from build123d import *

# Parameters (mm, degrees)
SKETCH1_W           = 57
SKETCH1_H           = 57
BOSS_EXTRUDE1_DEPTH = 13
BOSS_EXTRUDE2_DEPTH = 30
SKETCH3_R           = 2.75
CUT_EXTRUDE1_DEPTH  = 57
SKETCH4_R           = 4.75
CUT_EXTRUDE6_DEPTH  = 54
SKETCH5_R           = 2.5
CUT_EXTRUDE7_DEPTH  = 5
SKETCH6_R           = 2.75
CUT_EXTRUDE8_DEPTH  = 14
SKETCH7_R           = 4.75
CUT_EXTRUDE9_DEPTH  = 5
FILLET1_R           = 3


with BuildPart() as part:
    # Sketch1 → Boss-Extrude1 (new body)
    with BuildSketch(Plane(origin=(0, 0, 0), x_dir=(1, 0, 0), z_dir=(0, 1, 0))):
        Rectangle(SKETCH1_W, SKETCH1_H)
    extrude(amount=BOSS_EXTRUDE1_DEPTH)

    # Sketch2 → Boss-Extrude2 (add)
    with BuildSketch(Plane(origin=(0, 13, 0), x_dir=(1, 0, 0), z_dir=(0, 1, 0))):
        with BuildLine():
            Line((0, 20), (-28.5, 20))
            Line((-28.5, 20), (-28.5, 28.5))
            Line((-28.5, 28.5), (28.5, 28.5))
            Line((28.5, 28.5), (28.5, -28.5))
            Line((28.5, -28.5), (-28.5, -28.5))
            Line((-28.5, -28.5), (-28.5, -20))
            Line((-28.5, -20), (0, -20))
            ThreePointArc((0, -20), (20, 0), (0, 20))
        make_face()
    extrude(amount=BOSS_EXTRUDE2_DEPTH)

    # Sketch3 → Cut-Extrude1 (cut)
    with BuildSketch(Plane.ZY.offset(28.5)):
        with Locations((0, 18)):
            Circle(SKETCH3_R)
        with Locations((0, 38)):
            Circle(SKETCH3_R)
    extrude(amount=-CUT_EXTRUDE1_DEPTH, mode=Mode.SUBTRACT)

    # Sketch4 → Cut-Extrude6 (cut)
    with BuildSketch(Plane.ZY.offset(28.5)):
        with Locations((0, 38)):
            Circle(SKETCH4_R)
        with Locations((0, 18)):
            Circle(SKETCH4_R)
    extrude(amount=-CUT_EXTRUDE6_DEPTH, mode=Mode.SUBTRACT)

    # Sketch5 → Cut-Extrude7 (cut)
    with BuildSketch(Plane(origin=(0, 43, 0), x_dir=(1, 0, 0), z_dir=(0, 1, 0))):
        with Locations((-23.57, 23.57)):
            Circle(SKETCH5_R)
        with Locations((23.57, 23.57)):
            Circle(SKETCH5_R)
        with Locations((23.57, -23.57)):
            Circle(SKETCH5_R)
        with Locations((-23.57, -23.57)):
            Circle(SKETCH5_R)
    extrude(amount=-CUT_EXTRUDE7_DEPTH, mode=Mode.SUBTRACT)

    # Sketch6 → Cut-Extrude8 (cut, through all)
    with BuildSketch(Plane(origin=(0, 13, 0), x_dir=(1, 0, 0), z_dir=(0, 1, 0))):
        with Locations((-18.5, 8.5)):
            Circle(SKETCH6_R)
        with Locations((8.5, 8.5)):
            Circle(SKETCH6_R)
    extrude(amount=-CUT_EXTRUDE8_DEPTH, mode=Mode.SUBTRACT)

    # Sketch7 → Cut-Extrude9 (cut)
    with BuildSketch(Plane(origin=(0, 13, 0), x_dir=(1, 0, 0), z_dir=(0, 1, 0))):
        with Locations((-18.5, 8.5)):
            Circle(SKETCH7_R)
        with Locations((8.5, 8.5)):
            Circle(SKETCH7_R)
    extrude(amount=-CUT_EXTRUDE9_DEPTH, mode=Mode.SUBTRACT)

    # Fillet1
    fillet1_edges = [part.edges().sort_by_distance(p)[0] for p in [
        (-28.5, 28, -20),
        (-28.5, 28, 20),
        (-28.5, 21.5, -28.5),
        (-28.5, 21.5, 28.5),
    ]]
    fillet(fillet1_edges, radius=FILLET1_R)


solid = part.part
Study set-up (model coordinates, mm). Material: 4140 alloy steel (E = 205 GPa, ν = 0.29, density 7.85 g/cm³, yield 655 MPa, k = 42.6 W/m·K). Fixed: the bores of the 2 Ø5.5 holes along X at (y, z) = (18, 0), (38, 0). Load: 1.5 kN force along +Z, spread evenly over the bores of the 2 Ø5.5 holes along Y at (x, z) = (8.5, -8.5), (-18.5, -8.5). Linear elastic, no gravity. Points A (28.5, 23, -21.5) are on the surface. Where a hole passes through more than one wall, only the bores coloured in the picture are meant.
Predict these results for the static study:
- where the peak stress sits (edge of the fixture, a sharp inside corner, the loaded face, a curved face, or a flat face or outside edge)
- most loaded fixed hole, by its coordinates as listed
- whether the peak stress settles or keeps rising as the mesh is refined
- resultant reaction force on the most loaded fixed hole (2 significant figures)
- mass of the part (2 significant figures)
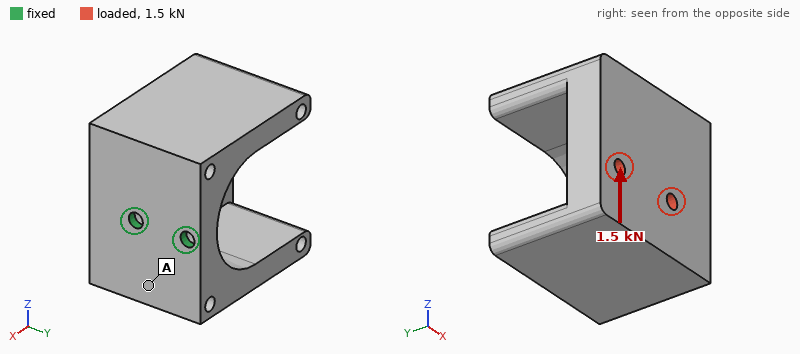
edge of the fixture
(18, 0)
keeps rising
2.2 kN
660 g
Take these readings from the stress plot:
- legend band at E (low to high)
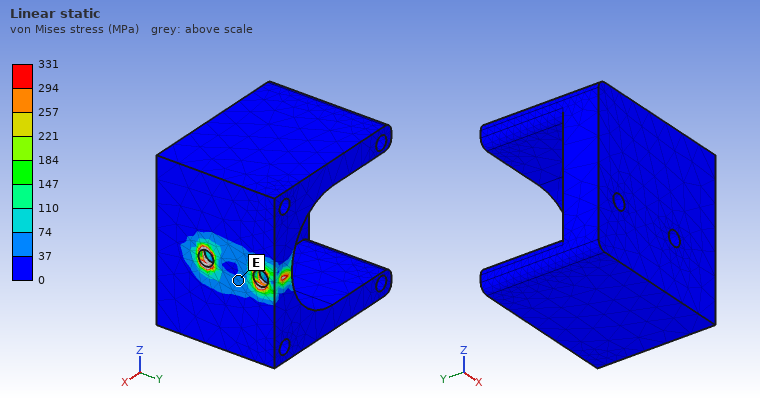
37 to 74 MPa
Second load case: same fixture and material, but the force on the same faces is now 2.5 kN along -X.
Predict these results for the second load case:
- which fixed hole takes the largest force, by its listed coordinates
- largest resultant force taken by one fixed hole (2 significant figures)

(18, 0)
3.9 kN
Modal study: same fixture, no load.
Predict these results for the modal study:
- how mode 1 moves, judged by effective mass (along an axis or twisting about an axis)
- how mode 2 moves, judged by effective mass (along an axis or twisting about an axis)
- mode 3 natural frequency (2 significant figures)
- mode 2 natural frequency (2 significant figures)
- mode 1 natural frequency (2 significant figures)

along Z
along Y
4500 Hz
2200 Hz
780 Hz
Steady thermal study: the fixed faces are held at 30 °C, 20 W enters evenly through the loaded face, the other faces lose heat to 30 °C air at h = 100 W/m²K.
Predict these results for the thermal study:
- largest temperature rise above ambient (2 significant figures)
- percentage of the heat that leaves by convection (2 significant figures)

20 K
70 %
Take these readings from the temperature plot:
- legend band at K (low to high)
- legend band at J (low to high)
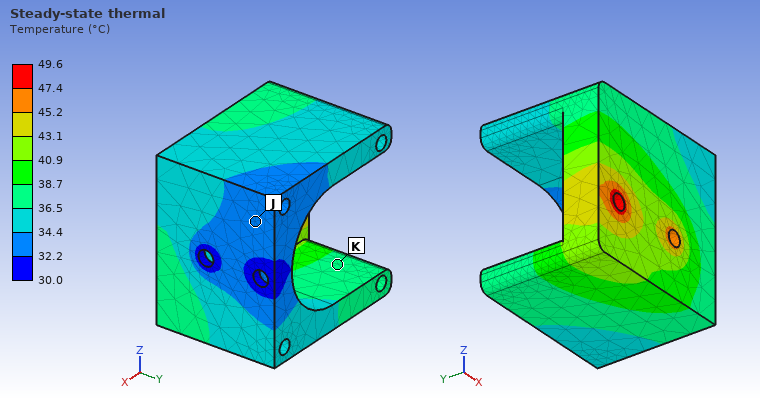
36.5 to 38.7 °C
32.2 to 34.4 °C
